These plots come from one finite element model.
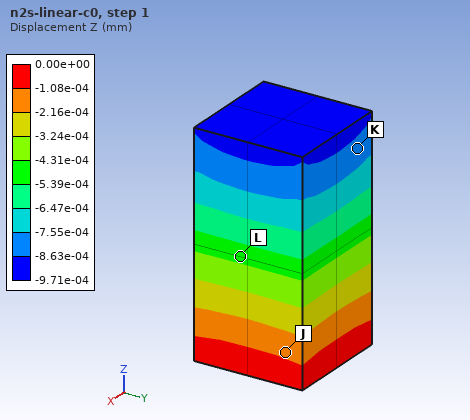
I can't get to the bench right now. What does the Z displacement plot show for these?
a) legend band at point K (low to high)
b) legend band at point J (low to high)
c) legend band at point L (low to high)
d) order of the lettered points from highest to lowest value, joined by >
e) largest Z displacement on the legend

-8.63e-04 to -7.55e-04 mm
-2.16e-04 to -1.08e-04 mm
-5.39e-04 to -4.31e-04 mm
J > L > K
0.00e+00 mm
